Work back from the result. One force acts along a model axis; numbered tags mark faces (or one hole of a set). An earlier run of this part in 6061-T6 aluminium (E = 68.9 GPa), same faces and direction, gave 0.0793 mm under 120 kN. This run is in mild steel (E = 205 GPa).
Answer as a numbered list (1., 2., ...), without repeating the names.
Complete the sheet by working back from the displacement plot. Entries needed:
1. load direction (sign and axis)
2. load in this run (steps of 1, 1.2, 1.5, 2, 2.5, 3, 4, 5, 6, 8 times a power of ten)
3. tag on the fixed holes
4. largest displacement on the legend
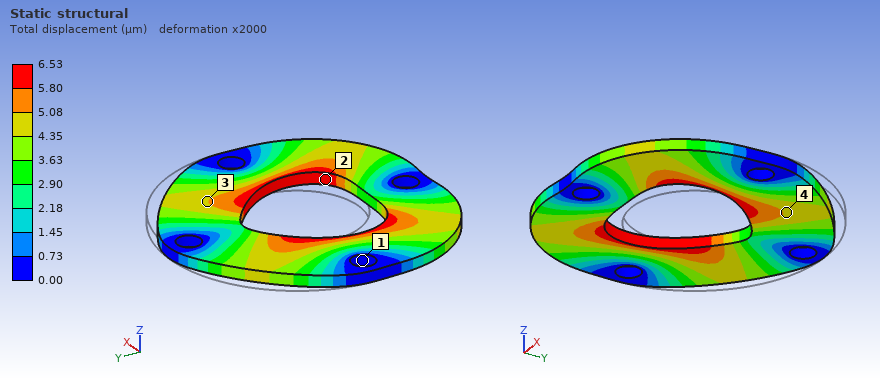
1. -Y
2. 30 kN
3. 1
4. 6.53 µm
